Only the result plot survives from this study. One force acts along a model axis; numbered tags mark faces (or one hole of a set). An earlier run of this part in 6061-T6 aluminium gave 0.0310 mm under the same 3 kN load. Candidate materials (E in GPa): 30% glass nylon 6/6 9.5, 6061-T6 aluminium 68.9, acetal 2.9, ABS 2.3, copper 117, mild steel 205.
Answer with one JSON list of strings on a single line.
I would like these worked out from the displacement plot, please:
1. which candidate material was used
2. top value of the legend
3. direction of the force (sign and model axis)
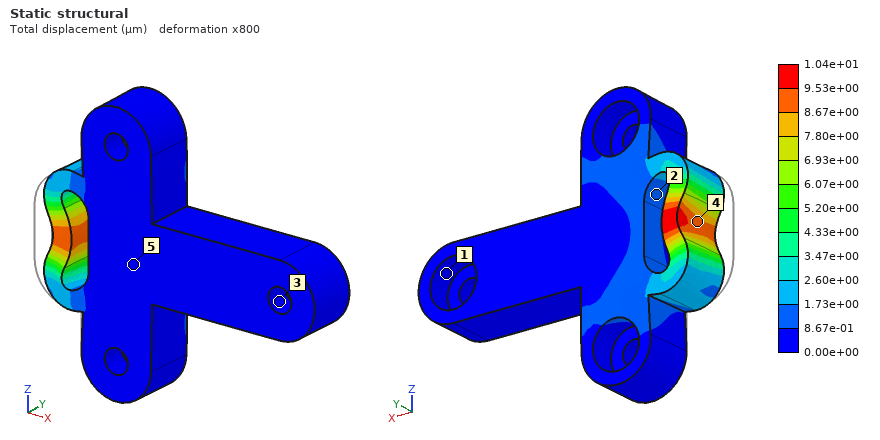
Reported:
["mild steel", "1.04e+01 µm", "+X"]
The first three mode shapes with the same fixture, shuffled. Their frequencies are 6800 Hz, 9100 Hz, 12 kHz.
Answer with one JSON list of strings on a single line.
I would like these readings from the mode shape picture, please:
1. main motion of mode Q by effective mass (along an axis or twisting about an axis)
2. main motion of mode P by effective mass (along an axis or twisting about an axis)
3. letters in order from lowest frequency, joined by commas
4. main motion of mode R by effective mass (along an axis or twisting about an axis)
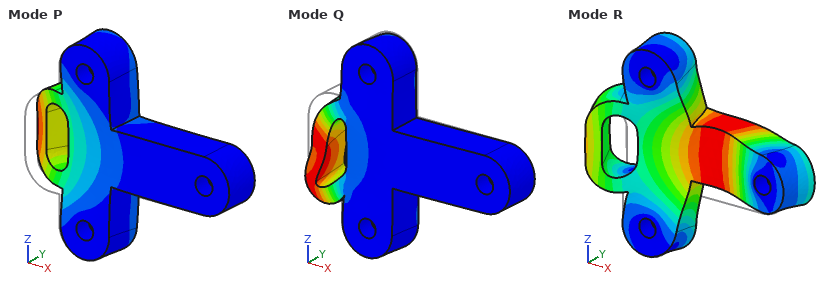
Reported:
["along Z", "along Y", "P, R, Q", "along Y"]
